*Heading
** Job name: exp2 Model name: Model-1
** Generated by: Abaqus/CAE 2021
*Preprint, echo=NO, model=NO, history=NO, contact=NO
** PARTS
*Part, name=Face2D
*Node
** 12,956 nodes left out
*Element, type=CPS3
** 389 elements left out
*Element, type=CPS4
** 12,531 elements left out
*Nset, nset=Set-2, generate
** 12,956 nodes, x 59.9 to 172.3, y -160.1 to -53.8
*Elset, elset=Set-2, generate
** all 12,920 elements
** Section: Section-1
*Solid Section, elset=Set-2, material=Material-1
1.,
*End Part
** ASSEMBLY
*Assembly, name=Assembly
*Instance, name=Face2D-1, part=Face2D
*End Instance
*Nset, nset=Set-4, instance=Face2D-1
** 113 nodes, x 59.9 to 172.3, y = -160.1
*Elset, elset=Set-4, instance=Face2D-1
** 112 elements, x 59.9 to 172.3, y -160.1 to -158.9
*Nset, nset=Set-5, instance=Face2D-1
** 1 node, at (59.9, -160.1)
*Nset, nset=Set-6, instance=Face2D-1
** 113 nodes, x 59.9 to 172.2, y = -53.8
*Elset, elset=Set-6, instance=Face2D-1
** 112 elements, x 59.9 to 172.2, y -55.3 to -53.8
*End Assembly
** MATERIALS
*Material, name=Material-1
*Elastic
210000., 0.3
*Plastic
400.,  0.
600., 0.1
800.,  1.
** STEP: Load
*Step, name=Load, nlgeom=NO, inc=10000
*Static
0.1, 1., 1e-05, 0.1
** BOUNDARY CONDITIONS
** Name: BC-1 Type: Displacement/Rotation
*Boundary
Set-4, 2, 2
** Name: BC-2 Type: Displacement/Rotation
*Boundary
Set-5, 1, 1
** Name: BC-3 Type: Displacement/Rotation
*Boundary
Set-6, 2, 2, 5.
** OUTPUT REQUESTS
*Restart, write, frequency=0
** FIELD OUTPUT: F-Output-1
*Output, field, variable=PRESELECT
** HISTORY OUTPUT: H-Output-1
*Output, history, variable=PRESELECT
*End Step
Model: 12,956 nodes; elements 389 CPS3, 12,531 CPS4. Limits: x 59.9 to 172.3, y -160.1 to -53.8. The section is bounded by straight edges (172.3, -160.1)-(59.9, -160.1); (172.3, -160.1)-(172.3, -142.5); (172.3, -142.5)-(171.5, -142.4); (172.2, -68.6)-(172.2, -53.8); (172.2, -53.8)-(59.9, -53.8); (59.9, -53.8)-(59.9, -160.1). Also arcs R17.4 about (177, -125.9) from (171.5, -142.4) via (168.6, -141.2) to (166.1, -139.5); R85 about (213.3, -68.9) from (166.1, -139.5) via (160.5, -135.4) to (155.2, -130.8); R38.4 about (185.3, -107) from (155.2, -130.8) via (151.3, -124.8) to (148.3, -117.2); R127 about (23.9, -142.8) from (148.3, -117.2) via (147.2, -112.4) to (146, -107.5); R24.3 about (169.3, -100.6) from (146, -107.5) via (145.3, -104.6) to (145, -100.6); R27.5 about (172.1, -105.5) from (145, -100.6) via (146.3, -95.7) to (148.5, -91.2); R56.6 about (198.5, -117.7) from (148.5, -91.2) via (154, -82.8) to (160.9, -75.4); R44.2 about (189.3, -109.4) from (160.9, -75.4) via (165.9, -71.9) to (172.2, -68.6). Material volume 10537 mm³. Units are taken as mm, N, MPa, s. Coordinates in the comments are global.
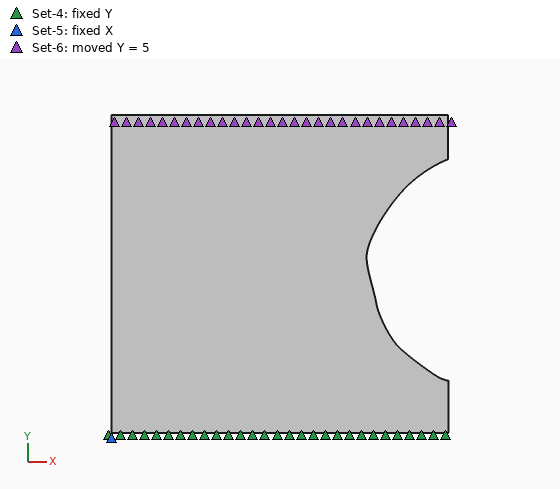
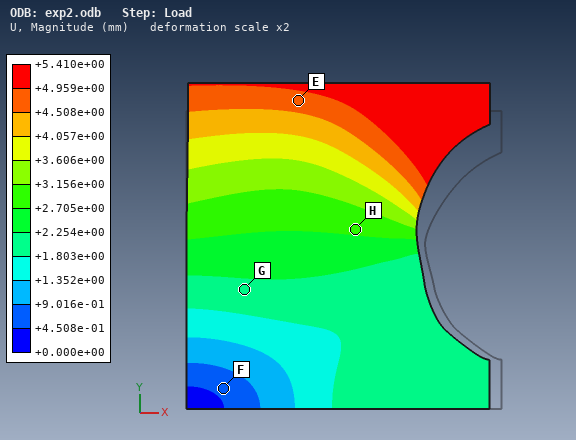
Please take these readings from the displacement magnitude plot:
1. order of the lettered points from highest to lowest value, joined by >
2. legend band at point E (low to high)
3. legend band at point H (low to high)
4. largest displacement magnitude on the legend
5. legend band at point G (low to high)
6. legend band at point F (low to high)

E > H > G > F
+4.508e+00 to +4.959e+00 mm
+2.705e+00 to +3.156e+00 mm
+5.410e+00 mm
+1.803e+00 to +2.254e+00 mm
+4.508e-01 to +9.016e-01 mm
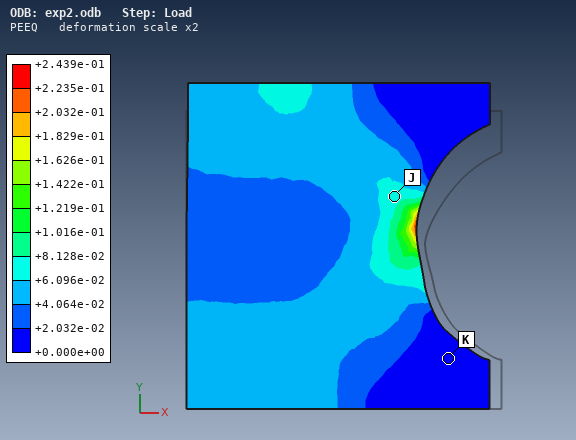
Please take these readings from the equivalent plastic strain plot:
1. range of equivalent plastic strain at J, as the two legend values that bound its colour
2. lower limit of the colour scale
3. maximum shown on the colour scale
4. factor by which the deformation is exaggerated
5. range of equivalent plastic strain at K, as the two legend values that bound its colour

+6.096e-02 to +8.128e-02
+0.000e+00
+2.439e-01
2
+0.000e+00 to +2.032e-02
